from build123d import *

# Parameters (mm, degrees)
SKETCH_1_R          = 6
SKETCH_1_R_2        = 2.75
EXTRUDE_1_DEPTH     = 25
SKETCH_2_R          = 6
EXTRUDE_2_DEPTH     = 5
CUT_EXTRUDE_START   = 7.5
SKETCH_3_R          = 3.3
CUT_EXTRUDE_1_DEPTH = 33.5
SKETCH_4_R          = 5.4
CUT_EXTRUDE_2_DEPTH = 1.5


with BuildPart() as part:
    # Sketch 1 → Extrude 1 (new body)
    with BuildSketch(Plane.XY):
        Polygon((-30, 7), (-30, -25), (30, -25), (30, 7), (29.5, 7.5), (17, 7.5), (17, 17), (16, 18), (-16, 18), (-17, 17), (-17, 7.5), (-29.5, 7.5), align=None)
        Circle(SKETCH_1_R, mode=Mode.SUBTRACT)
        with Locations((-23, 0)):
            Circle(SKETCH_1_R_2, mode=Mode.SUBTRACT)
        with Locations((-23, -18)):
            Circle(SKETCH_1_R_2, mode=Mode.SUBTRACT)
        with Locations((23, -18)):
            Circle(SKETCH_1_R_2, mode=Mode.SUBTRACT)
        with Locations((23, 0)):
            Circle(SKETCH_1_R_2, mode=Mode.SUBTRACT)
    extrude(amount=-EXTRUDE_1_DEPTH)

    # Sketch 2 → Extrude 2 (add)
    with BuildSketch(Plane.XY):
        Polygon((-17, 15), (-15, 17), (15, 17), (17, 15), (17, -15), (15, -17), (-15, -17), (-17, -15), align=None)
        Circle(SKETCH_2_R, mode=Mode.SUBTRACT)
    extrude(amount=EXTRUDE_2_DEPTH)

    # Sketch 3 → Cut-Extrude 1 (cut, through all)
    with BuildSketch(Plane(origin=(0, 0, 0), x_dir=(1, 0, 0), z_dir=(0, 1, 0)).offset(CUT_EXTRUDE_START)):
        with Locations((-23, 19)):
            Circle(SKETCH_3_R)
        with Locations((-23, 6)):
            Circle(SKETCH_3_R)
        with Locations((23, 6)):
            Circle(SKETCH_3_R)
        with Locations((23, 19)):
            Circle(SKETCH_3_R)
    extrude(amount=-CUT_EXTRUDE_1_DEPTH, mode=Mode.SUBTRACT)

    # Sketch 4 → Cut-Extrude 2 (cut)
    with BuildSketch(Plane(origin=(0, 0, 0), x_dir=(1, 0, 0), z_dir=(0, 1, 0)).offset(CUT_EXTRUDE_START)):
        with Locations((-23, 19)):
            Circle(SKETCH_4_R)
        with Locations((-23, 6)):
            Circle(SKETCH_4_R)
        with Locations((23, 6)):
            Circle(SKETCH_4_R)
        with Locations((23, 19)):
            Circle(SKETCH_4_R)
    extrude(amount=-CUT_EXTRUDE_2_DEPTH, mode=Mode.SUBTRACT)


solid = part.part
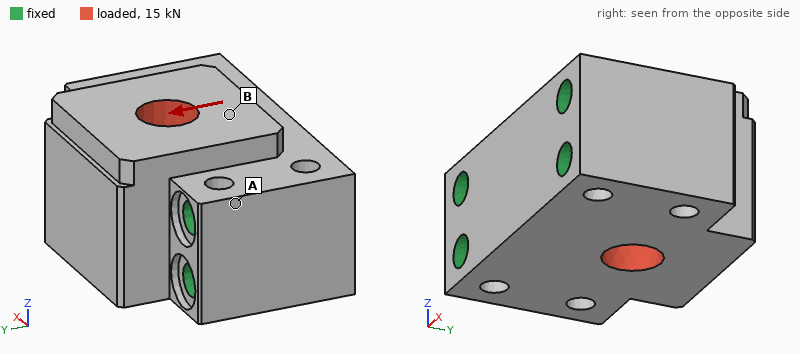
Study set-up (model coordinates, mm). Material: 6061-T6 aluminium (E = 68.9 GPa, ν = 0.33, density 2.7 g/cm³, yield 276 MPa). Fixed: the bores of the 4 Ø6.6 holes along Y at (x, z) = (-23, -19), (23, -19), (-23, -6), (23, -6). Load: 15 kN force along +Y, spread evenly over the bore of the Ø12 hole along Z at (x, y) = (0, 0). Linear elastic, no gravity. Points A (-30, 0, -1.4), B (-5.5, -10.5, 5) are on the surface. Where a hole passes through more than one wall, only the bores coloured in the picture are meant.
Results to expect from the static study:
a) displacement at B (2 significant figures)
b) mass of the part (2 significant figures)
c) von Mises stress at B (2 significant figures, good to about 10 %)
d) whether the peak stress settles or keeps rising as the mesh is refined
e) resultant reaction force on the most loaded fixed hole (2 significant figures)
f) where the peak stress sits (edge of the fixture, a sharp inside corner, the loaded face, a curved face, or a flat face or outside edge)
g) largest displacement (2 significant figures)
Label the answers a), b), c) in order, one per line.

a) 7.0 µm
b) 150 g
c) 11 MPa
d) keeps rising
e) 4.5 kN
f) edge of the fixture
g) 9.8 µm
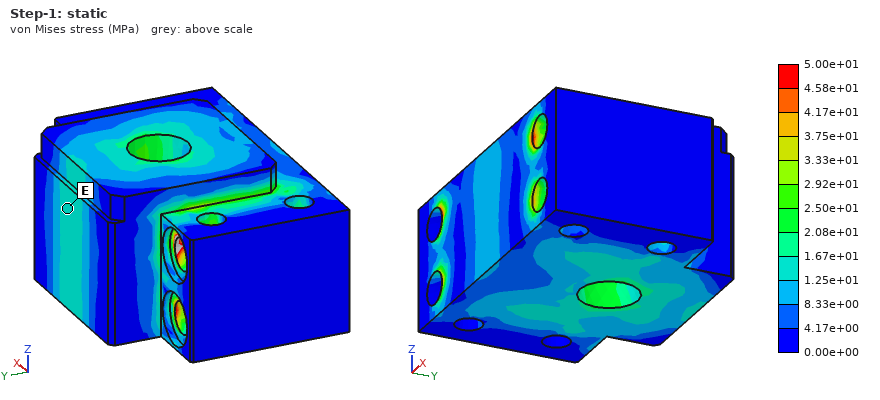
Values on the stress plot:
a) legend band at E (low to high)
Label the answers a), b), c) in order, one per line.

a) 1.25e+01 to 1.67e+01 MPa
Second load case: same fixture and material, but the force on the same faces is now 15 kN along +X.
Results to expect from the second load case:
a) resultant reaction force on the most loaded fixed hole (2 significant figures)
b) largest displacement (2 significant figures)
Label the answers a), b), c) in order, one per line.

a) 4.2 kN
b) 5.5 µm
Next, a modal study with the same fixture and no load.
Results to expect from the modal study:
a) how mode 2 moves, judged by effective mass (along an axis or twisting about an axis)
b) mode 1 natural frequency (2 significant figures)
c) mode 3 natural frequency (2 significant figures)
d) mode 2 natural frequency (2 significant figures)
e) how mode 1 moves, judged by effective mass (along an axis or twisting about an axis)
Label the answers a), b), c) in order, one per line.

a) along Y
b) 19 kHz
c) 31 kHz
d) 29 kHz
e) along Z
